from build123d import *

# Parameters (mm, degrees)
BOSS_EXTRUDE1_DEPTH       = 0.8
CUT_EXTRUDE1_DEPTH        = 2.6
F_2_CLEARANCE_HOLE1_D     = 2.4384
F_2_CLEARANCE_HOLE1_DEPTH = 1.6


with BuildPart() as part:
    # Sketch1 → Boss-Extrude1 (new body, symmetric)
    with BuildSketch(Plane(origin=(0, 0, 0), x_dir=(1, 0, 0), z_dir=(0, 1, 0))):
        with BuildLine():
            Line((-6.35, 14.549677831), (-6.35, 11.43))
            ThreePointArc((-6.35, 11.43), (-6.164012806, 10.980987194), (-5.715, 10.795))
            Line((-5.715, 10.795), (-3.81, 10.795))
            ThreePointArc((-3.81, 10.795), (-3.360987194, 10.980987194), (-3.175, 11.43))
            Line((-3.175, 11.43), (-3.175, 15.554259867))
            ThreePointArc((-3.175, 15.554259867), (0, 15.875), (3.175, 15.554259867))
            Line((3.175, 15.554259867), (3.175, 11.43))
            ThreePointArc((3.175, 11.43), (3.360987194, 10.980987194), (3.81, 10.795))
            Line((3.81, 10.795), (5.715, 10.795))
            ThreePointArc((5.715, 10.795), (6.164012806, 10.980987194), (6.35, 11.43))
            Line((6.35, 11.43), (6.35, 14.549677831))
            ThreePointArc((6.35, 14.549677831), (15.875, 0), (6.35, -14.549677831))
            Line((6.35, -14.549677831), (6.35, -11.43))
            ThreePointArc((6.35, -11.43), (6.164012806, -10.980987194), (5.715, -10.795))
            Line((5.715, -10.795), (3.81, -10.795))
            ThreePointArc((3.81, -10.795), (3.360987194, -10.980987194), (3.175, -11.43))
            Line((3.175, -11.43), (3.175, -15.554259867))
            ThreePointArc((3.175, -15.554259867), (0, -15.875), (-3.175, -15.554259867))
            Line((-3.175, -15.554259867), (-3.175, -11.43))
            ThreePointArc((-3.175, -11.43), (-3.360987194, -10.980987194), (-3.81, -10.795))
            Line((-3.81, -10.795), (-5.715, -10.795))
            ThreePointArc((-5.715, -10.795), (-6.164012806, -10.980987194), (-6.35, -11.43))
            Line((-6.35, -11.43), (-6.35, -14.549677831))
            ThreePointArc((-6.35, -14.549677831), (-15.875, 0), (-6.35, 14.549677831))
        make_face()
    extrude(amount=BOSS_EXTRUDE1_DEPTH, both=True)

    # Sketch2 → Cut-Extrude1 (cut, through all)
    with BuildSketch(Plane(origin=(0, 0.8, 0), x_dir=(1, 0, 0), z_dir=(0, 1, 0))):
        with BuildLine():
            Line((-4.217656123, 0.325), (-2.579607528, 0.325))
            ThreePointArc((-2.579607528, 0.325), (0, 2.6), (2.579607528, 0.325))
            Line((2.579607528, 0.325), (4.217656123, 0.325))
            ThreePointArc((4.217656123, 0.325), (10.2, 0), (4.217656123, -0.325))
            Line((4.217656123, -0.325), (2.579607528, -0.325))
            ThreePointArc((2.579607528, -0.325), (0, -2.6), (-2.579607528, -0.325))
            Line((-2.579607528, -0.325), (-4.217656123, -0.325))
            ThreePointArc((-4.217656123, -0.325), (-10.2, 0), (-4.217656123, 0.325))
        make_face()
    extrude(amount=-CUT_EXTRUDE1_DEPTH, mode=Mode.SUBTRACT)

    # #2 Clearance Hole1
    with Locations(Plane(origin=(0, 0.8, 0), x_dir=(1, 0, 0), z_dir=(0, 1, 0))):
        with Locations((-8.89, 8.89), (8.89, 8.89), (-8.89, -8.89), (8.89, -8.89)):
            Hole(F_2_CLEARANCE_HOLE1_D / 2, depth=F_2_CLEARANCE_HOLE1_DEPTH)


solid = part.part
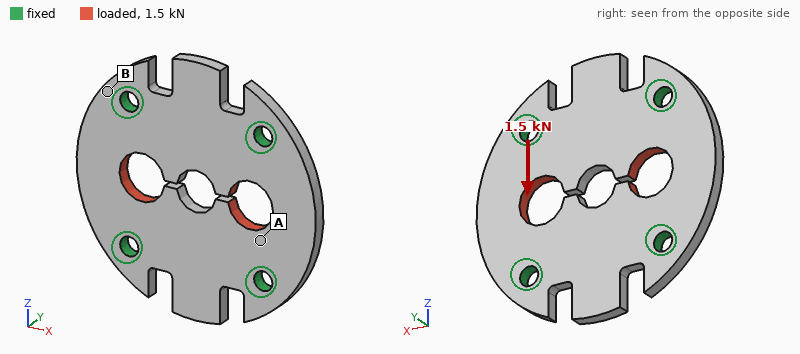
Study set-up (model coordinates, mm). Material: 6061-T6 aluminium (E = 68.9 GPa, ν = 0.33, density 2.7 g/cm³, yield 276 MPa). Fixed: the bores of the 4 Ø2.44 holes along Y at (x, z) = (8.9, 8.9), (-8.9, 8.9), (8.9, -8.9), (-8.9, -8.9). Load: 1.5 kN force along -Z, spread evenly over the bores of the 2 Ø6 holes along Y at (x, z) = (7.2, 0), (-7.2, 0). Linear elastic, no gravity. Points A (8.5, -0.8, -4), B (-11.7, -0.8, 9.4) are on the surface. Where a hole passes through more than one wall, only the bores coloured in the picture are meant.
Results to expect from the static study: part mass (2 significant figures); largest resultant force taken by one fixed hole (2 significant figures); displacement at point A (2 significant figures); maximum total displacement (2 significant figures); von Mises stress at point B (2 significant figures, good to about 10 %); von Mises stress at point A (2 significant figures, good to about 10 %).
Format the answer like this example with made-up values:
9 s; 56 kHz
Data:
2.8 g; 380 N; 2.2 µm; 4.9 µm; 13 MPa; 33 MPa
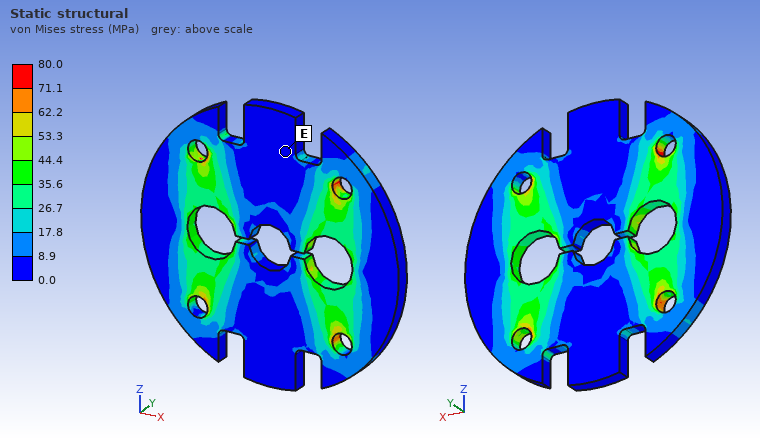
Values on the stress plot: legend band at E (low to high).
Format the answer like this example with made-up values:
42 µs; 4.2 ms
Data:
0.0 to 8.9 MPa
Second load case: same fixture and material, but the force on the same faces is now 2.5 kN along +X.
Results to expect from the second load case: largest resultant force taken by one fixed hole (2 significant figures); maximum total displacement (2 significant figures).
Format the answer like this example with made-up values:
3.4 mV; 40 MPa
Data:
630 N; 11 µm
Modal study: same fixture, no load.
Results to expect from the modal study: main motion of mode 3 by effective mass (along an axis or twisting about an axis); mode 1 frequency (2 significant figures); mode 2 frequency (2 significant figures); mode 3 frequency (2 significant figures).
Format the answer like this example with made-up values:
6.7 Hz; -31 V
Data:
along Y; 16 kHz; 16 kHz; 19 kHz
